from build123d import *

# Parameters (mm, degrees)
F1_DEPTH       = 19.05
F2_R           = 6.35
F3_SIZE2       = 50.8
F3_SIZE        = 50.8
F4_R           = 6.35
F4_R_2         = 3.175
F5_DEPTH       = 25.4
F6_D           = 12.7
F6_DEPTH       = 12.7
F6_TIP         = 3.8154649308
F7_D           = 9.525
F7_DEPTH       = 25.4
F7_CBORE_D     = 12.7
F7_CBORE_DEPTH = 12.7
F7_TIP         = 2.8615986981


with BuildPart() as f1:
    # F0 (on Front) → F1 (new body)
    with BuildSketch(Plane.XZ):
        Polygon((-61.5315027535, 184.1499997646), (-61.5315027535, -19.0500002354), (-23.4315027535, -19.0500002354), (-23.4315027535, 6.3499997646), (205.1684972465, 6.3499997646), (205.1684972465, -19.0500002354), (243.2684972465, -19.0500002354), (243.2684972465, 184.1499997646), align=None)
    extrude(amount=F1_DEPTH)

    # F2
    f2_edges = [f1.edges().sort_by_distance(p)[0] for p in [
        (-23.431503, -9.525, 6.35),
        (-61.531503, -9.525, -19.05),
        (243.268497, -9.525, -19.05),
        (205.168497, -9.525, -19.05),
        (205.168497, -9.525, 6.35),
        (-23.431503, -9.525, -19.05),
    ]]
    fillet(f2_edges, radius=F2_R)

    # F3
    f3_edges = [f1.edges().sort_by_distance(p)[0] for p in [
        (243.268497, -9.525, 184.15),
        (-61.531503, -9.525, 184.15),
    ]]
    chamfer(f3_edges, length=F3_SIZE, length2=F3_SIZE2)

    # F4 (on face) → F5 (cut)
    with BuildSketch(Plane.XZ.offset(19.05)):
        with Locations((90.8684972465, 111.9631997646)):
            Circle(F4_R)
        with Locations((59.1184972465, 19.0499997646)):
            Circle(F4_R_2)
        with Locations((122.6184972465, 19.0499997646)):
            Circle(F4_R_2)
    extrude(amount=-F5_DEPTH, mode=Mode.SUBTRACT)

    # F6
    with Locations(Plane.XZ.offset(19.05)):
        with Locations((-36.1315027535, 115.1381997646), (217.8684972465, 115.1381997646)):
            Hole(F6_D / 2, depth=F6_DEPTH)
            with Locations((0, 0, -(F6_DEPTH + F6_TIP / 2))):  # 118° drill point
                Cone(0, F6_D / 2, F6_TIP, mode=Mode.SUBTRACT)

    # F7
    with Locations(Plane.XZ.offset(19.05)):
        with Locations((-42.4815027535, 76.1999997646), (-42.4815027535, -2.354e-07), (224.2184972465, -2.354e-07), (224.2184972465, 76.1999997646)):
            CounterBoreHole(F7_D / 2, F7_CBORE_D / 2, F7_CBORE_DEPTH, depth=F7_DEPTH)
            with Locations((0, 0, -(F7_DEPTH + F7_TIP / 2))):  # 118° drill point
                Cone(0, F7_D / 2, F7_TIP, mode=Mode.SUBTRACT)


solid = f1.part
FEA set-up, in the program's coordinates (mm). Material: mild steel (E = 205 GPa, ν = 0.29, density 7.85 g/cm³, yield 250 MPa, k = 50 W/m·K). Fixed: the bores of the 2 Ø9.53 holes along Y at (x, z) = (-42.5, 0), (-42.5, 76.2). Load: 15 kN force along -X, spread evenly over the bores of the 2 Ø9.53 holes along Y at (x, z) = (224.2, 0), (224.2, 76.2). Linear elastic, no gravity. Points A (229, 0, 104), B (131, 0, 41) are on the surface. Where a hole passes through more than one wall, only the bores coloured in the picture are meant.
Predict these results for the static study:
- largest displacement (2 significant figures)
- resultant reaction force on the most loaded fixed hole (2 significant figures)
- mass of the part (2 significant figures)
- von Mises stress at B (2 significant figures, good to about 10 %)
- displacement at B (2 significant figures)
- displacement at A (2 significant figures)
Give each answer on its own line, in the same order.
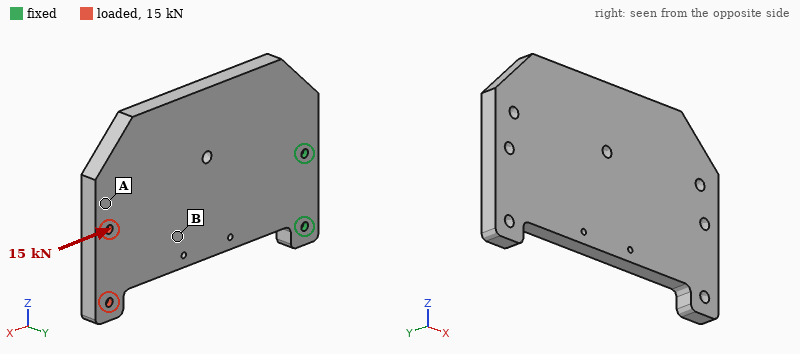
0.23 mm
7.7 kN
7.9 kg
20 MPa
0.086 mm
0.20 mm
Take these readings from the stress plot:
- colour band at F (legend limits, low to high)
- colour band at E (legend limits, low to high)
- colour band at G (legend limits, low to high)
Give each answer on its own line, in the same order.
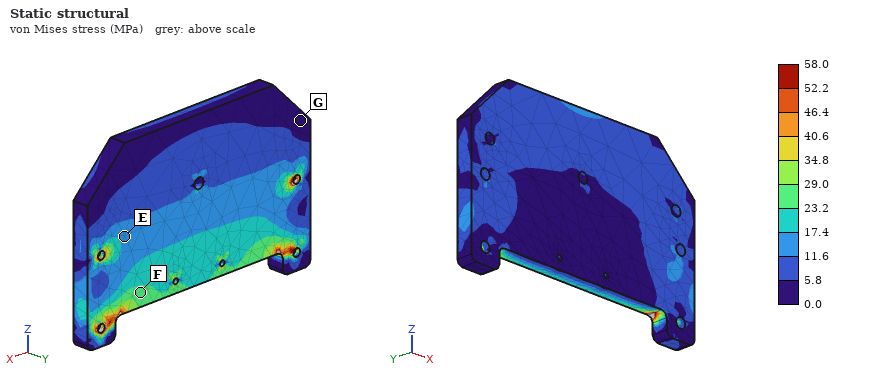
23.2 to 29.0 MPa
11.6 to 17.4 MPa
0.0 to 5.8 MPa
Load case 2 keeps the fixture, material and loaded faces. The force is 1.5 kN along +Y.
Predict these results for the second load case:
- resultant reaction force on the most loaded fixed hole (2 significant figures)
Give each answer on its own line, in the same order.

2.0 kN
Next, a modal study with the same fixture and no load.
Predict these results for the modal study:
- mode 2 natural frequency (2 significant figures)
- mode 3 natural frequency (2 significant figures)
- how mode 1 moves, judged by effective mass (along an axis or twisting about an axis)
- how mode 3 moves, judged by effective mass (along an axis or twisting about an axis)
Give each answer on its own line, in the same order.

470 Hz
610 Hz
along Y
along Z
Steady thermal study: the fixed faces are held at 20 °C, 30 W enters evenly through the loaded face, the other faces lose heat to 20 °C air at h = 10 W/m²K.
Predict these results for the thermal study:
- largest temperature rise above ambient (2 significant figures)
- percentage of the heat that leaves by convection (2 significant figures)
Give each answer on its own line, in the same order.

50 K
67 %
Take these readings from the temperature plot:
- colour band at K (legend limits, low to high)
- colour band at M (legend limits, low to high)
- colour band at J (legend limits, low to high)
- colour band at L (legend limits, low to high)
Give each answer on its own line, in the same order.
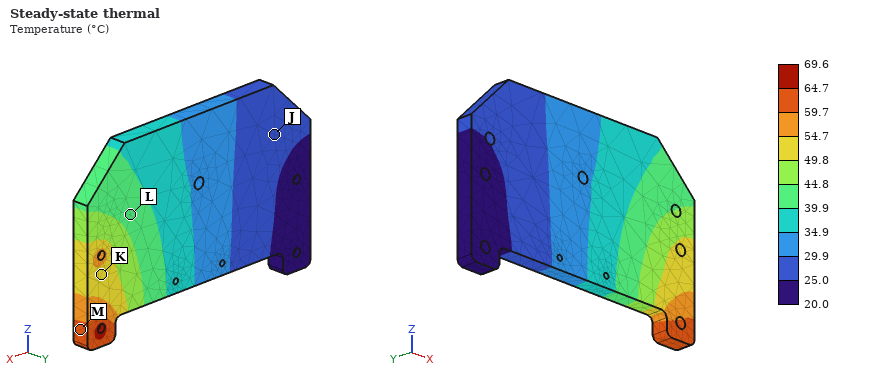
49.8 to 54.7 °C
59.7 to 64.7 °C
25.0 to 29.9 °C
39.9 to 44.8 °C
